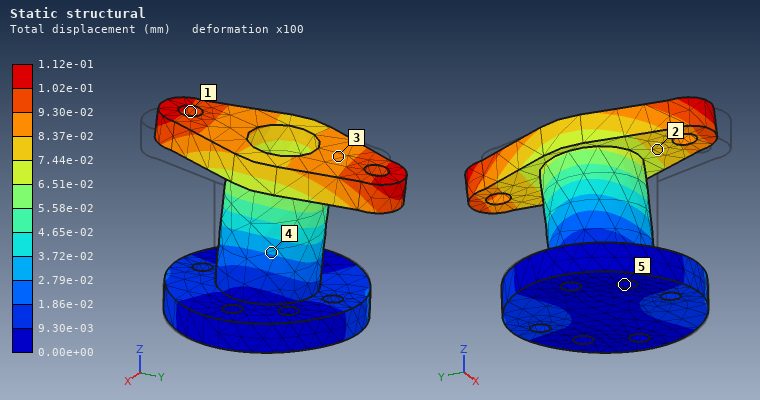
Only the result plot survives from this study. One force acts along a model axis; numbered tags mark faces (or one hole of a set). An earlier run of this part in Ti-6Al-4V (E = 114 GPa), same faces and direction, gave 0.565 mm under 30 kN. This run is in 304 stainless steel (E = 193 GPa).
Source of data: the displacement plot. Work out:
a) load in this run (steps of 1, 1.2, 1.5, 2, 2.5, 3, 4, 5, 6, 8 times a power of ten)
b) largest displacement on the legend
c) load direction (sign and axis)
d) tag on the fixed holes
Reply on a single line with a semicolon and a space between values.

10 kN; 1.12e-01 mm; +Y; 5
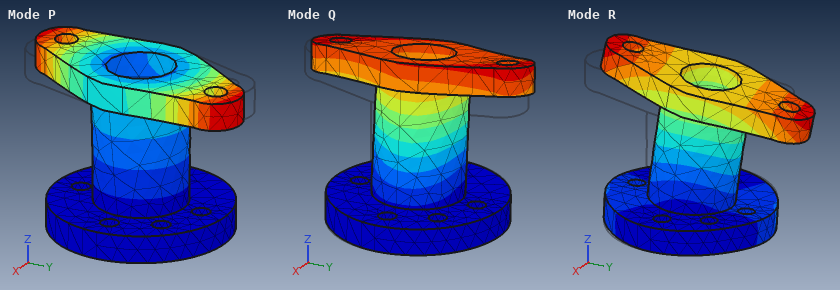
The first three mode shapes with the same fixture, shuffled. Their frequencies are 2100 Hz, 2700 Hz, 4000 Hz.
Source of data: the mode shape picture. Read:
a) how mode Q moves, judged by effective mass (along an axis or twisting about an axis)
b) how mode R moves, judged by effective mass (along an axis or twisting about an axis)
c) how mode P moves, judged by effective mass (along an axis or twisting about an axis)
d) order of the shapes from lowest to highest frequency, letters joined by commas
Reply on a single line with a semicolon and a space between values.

along X; along Y; twisting about Z; R, Q, P
